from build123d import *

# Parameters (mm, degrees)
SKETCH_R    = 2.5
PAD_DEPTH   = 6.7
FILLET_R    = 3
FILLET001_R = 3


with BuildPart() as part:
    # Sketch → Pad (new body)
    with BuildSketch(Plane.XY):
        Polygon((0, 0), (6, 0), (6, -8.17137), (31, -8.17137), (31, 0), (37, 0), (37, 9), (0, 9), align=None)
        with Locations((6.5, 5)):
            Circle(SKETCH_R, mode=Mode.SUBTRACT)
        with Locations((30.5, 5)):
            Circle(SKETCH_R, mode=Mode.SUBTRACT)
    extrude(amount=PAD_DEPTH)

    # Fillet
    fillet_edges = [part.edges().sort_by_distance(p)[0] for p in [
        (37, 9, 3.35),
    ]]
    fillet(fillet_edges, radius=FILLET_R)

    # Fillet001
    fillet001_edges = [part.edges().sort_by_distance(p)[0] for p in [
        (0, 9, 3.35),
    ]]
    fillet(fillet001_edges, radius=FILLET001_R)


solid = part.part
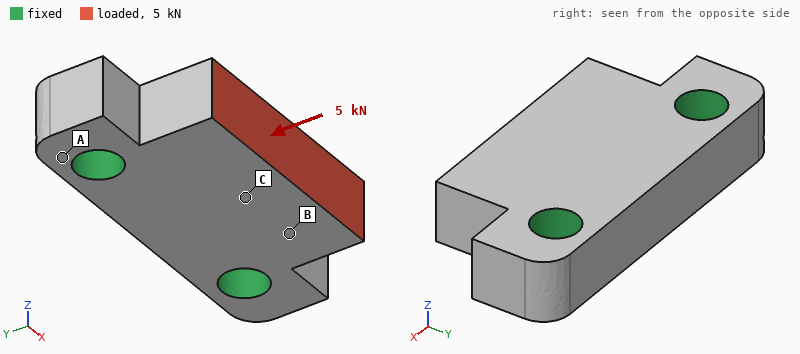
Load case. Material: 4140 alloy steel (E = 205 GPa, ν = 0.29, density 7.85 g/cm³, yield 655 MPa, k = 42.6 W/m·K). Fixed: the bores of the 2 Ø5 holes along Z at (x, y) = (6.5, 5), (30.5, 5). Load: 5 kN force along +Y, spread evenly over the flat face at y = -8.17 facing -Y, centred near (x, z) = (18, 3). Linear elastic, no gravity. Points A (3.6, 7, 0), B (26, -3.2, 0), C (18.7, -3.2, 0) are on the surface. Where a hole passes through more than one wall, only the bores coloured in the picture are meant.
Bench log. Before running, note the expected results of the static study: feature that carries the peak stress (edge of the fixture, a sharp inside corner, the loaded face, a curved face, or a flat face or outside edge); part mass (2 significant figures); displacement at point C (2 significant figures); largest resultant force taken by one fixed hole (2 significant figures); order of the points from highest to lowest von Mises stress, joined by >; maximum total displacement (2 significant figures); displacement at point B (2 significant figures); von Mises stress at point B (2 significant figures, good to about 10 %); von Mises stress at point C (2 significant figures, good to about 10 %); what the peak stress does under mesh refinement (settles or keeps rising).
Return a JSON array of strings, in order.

["edge of the fixture", "26 g", "2.5 µm", "2.6 kN", "B > C > A", "3.1 µm", "1.9 µm", "34 MPa", "20 MPa", "keeps rising"]
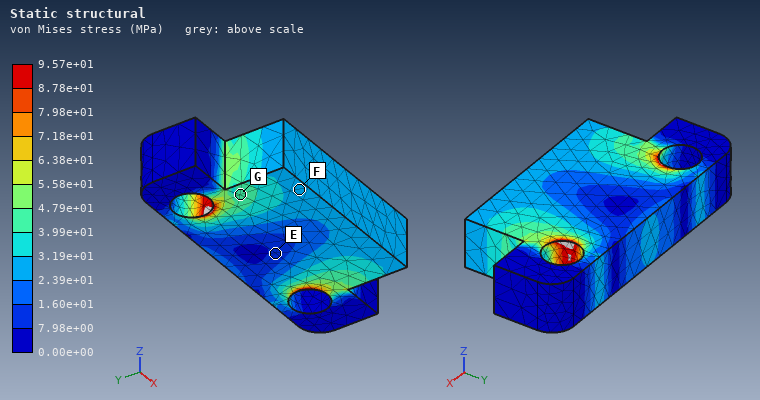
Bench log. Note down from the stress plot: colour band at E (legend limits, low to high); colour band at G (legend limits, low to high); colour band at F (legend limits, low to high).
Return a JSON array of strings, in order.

["7.98e+00 to 1.60e+01 MPa", "3.99e+01 to 4.79e+01 MPa", "2.39e+01 to 3.19e+01 MPa"]
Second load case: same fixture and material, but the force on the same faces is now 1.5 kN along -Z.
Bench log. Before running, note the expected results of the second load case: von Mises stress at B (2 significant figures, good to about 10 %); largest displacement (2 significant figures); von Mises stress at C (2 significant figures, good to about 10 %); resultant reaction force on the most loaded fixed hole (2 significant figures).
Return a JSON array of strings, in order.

["42 MPa", "13 µm", "38 MPa", "750 N"]
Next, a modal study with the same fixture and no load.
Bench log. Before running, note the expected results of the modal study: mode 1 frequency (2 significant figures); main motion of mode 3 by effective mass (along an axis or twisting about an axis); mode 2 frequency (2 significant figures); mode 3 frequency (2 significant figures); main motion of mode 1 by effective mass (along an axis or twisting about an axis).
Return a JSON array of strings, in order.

["25 kHz", "along Z", "44 kHz", "54 kHz", "along Z"]
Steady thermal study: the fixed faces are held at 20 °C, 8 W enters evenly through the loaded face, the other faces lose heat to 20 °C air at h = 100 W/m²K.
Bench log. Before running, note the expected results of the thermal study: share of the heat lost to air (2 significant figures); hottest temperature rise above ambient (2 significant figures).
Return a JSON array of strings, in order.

["8.9 %", "15 K"]
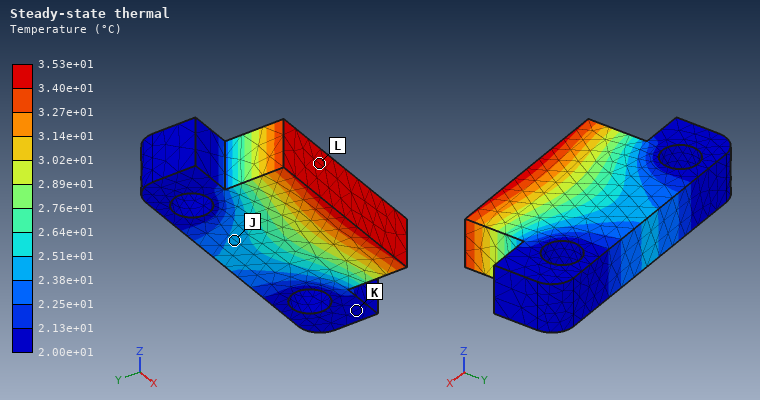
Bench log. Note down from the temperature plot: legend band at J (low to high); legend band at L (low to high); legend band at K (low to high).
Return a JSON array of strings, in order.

["2.38e+01 to 2.51e+01 °C", "3.40e+01 to 3.53e+01 °C", "2.00e+01 to 2.13e+01 °C"]
